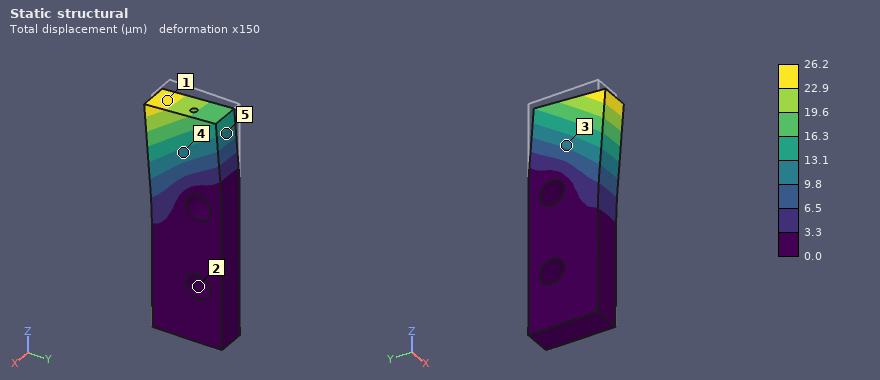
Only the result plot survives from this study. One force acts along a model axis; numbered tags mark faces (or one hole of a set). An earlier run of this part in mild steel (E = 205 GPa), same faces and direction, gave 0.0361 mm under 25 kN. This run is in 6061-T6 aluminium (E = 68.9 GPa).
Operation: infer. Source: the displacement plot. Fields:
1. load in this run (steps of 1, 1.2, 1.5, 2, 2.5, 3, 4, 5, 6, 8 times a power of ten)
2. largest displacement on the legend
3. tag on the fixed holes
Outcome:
6 kN
26.2 µm
2
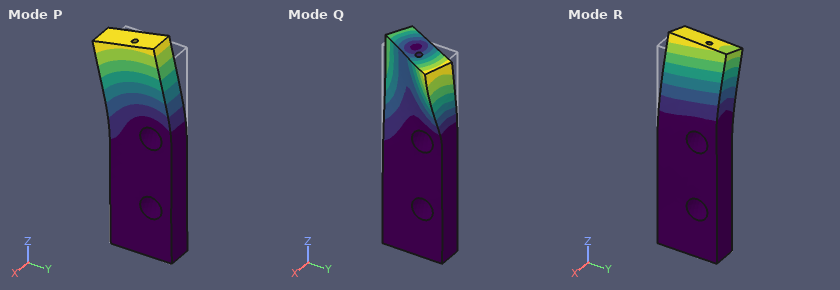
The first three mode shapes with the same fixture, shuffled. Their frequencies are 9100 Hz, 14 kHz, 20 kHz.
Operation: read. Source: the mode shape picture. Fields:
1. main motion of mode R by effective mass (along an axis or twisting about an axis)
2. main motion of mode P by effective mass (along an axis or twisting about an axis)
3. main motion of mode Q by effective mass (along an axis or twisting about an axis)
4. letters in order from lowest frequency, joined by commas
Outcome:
along X
along Y
twisting about Z
R, P, Q
